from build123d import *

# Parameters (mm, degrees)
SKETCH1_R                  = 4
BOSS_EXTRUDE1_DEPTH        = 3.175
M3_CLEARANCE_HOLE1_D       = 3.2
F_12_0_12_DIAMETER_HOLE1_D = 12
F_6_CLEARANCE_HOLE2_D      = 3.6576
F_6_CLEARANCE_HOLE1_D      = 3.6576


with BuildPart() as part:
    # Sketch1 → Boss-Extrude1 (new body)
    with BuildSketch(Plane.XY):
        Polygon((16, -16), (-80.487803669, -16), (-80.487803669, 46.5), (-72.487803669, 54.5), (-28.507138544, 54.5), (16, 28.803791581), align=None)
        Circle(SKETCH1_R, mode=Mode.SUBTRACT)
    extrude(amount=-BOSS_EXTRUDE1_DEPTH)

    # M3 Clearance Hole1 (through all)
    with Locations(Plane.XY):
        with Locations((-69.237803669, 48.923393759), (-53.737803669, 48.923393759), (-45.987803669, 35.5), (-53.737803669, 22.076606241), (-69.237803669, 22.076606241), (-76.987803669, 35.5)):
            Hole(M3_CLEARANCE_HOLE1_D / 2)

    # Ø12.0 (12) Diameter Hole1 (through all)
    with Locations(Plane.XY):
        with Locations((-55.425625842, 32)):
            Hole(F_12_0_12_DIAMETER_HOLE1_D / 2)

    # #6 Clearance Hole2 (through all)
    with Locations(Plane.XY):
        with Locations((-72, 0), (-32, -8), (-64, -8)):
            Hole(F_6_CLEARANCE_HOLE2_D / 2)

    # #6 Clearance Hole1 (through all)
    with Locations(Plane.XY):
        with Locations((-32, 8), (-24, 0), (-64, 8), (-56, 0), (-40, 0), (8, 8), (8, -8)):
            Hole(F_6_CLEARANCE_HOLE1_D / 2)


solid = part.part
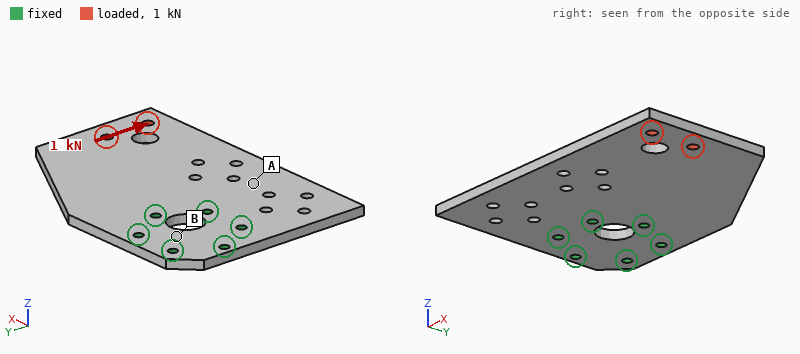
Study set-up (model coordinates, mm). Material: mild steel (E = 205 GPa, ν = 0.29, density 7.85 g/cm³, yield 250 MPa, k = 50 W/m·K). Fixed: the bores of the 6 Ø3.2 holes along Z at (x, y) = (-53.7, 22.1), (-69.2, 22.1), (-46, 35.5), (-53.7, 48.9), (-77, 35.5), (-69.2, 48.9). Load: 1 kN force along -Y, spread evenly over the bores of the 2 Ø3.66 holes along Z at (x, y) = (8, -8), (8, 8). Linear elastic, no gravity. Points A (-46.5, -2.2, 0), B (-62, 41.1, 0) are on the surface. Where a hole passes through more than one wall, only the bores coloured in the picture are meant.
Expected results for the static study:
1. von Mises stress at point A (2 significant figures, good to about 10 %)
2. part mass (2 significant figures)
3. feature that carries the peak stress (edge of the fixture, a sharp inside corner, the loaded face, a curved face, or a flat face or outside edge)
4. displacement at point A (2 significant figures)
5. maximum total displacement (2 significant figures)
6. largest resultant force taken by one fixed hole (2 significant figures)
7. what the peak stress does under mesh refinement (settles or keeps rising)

9.5 MPa
150 g
edge of the fixture
6.0 µm
22 µm
1.2 kN
keeps rising
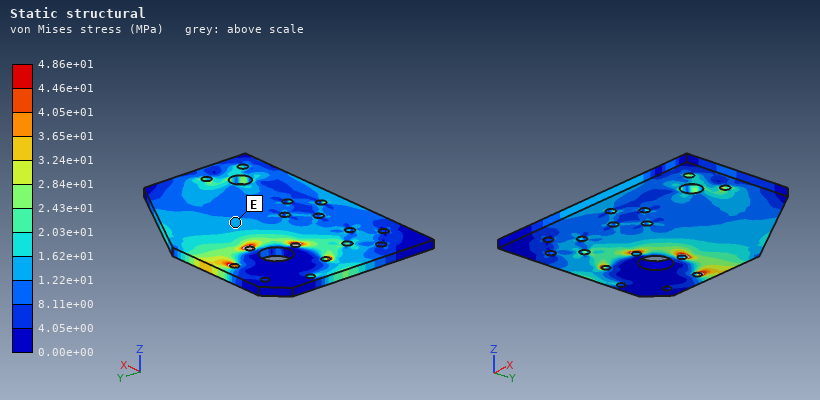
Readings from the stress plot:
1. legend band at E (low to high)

1.22e+01 to 1.62e+01 MPa
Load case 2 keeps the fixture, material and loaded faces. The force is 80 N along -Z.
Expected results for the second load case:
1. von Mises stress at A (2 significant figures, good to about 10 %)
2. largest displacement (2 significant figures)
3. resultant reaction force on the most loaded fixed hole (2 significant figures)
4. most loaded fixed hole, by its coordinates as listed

26 MPa
0.29 mm
130 N
(-46, 35.5)
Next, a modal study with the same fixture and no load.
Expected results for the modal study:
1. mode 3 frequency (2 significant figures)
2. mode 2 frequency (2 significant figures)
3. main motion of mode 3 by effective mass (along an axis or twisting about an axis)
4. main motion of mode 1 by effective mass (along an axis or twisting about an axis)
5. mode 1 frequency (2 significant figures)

2300 Hz
1400 Hz
along Z
along Z
590 Hz
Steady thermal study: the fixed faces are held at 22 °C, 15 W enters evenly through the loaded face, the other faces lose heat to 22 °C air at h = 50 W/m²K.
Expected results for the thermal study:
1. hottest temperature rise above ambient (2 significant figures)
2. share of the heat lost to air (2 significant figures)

77 K
73 %
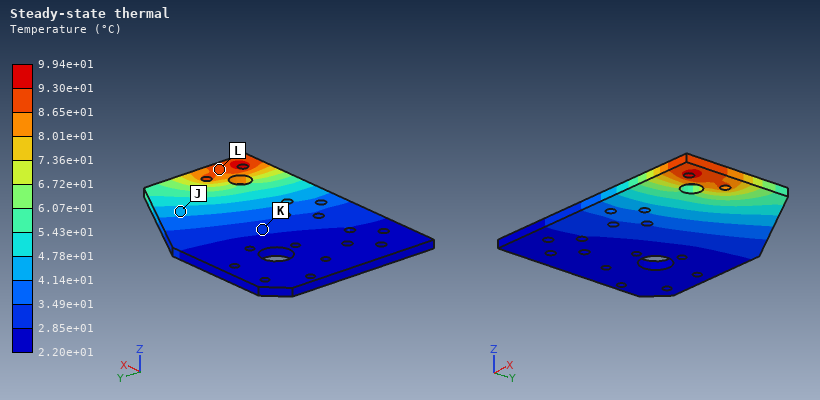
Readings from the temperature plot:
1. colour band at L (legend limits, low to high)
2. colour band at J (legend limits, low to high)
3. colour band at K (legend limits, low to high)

8.65e+01 to 9.30e+01 °C
4.14e+01 to 4.78e+01 °C
2.85e+01 to 3.49e+01 °C
